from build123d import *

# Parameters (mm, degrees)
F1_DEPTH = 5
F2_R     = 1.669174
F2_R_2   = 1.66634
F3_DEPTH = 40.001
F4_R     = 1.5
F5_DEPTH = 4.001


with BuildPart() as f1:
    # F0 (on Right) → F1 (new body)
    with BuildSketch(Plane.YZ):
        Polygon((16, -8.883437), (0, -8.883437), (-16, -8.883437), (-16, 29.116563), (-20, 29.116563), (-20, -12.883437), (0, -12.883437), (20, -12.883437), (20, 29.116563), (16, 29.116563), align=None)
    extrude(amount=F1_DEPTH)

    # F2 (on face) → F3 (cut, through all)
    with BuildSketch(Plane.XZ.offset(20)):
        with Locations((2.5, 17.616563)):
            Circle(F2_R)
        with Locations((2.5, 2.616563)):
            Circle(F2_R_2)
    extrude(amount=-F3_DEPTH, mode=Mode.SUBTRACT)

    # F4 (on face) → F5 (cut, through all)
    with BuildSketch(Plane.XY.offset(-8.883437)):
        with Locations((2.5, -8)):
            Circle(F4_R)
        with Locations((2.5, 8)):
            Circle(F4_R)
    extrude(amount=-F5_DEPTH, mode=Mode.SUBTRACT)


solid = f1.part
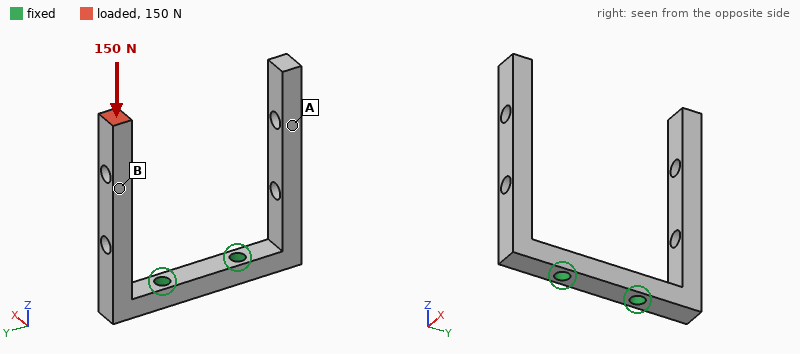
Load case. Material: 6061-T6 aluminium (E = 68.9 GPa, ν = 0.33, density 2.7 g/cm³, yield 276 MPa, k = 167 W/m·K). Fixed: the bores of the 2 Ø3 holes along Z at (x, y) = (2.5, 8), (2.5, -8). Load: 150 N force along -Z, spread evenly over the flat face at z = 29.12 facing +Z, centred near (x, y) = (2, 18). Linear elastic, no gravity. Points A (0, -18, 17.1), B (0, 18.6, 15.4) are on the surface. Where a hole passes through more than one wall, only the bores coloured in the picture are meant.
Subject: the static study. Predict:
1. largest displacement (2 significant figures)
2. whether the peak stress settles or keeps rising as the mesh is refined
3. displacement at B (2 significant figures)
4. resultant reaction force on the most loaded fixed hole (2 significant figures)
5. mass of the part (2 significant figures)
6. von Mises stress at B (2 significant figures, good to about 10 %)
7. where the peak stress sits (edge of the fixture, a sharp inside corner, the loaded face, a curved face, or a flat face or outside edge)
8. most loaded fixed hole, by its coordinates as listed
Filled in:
0.14 mm
keeps rising
0.095 mm
150 N
5.7 g
19 MPa
edge of the fixture
(2.5, 8)
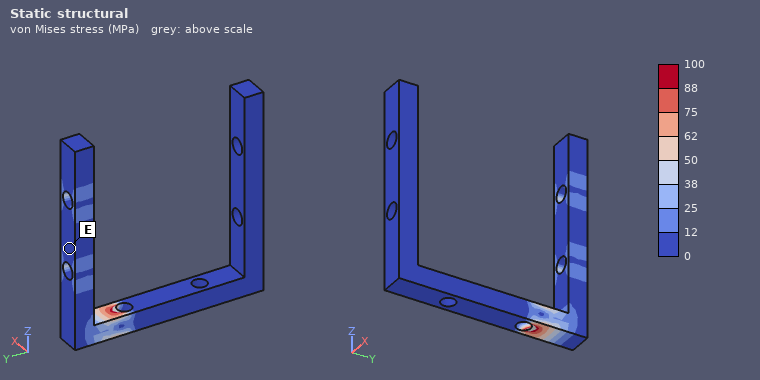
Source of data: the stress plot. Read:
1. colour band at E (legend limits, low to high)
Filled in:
0 to 12 MPa
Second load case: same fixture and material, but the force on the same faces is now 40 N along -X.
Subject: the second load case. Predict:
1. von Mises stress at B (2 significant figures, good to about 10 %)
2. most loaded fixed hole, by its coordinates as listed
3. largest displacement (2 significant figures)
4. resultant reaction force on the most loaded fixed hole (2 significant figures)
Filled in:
47 MPa
(2.5, 8)
0.66 mm
42 N
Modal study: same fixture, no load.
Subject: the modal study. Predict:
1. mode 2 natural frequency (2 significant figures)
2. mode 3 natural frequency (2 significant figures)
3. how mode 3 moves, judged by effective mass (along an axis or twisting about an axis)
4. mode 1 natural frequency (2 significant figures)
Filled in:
1500 Hz
1600 Hz
along X
1500 Hz
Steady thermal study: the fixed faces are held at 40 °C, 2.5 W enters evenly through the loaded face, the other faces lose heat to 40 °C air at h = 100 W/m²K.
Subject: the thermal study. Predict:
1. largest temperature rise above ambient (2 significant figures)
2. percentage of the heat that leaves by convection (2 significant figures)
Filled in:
30 K
47 %
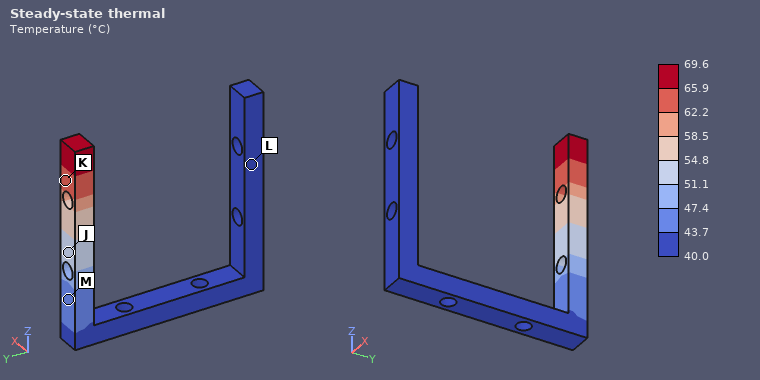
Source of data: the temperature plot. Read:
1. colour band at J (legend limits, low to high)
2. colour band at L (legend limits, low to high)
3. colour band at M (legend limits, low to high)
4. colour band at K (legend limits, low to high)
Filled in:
51.1 to 54.8 °C
40.0 to 43.7 °C
43.7 to 47.4 °C
62.2 to 65.9 °C
